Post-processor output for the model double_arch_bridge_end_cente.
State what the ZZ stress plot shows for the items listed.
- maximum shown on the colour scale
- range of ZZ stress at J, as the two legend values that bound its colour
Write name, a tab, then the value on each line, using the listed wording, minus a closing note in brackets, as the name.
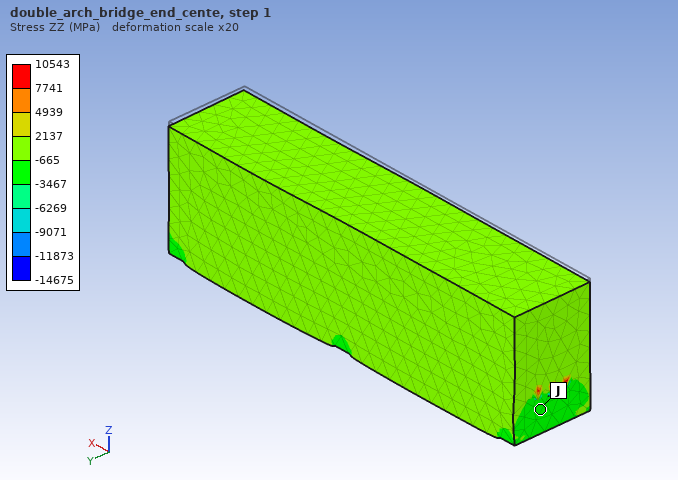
maximum shown on the colour scale	10543 MPa
range of ZZ stress at J, as the two legend values that bound its colour	-3467 to -665 MPa
